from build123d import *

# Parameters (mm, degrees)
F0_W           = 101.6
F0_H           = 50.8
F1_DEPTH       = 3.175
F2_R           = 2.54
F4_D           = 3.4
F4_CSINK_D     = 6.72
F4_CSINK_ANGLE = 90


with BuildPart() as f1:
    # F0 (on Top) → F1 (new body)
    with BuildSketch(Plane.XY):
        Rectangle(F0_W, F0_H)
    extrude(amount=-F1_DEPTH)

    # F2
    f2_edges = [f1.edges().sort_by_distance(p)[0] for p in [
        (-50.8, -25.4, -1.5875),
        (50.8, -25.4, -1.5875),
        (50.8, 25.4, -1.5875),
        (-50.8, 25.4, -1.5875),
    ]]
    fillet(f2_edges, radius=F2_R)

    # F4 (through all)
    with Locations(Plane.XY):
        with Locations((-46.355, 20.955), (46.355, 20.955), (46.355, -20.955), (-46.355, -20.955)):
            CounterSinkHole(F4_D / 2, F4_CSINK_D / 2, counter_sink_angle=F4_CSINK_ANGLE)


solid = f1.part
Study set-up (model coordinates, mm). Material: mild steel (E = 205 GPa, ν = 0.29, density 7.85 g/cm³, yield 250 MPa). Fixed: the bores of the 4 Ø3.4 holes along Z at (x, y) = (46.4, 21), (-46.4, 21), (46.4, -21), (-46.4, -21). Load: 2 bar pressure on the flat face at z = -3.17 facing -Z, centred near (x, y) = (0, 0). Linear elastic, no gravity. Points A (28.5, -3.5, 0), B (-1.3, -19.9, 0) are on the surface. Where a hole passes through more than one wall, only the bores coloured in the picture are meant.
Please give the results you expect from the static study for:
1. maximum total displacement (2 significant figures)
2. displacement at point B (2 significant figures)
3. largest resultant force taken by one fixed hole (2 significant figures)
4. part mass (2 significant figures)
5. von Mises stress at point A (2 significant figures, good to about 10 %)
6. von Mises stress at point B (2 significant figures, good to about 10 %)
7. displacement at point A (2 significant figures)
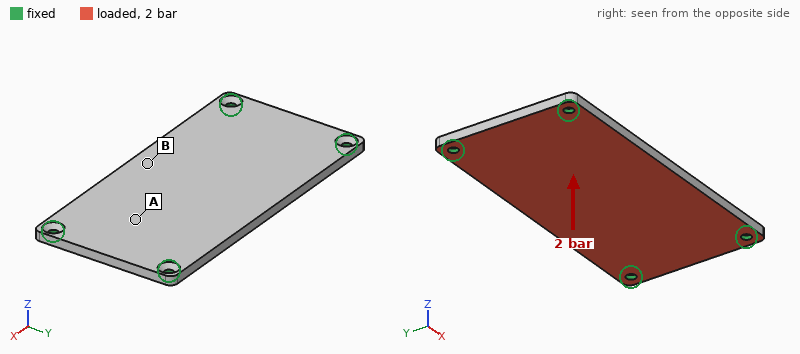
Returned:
0.12 mm
0.12 mm
460 N
130 g
17 MPa
61 MPa
0.060 mm
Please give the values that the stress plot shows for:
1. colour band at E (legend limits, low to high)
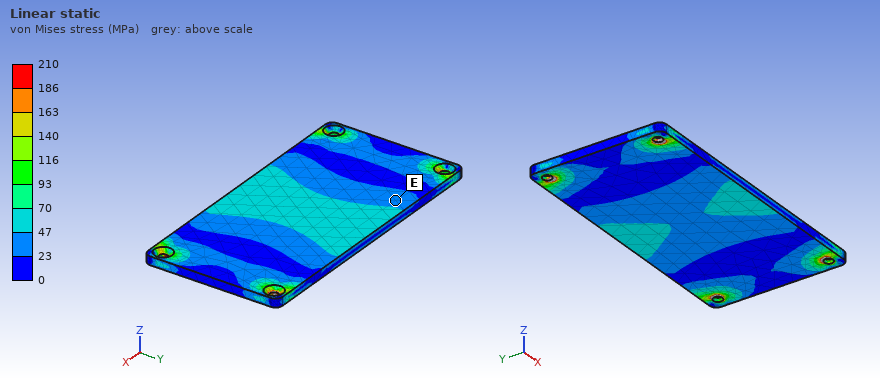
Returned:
23 to 47 MPa
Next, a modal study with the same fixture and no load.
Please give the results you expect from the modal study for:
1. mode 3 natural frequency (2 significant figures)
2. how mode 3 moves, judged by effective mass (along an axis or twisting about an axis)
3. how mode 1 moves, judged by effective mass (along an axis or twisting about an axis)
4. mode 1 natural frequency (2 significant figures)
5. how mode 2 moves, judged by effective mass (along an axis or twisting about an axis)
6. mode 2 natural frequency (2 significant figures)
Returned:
4200 Hz
twisting about Y
along Z
1500 Hz
twisting about X
2800 Hz
